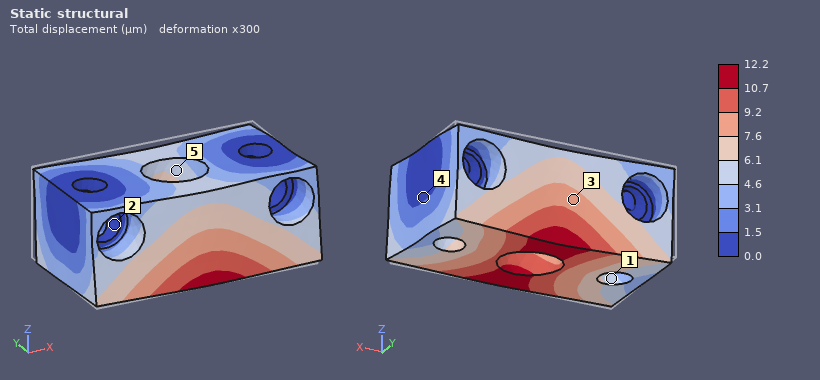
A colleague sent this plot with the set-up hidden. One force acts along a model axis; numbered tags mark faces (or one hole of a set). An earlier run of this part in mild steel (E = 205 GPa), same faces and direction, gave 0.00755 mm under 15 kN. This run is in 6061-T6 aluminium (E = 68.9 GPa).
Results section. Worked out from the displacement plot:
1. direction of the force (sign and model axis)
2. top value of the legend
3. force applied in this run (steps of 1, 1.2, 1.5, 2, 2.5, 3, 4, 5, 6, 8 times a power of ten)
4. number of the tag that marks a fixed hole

-Y
12.2 µm
8 kN
2
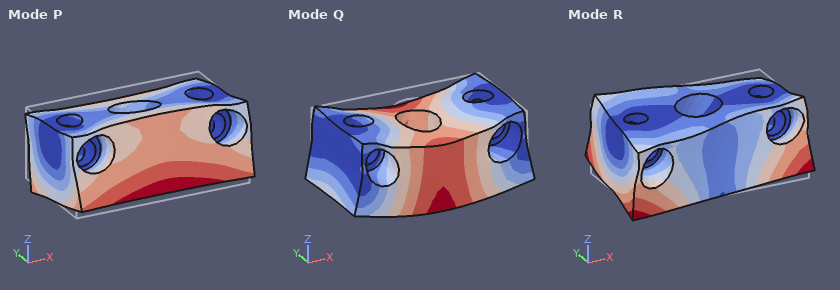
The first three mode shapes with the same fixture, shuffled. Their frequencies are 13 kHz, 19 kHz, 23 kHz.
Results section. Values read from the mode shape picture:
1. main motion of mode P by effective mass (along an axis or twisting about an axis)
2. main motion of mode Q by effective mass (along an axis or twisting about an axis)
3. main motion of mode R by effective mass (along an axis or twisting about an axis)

along Y
along Z
twisting about Z
